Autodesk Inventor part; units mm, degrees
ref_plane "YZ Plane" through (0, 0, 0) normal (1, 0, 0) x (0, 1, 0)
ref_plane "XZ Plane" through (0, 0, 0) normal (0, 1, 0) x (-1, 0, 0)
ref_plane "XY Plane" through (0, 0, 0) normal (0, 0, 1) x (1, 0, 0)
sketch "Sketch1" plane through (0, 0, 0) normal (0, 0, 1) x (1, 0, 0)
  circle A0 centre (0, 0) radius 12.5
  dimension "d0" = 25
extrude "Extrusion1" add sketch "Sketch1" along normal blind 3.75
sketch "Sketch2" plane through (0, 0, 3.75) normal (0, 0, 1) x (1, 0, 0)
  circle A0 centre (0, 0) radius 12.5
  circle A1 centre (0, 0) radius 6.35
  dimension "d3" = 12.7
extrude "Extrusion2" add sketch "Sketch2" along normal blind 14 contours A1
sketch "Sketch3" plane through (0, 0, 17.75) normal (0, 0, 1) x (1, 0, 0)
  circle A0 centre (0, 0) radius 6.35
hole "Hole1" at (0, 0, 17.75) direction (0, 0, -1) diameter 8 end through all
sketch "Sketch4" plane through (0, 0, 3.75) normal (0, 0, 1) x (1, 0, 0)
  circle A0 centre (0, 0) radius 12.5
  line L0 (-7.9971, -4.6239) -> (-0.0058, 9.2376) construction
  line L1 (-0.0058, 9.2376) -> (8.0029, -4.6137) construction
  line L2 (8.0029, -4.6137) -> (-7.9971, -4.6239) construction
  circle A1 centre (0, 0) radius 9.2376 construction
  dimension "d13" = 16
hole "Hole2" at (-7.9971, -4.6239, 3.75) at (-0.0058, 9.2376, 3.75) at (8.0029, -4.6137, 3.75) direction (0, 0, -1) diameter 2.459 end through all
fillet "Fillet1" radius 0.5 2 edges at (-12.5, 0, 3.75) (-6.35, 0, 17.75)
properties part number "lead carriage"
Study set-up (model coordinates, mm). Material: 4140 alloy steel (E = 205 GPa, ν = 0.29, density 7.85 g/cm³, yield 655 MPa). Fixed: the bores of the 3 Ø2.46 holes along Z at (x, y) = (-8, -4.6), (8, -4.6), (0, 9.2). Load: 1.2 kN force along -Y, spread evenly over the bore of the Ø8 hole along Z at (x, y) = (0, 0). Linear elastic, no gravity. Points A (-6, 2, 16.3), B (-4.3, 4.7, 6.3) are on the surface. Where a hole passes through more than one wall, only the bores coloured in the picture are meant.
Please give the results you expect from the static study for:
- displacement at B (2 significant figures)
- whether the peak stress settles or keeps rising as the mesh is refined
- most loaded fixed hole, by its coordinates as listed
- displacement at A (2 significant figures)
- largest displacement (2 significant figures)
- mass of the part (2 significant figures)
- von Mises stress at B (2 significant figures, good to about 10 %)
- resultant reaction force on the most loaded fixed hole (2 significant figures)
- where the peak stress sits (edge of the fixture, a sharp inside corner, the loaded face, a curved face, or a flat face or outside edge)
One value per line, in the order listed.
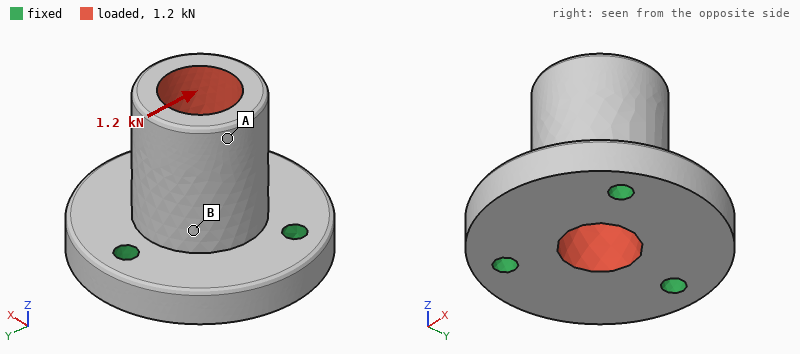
2.4 µm
keeps rising
(0, 9.2)
6.7 µm
7.9 µm
21 g
27 MPa
730 N
edge of the fixture
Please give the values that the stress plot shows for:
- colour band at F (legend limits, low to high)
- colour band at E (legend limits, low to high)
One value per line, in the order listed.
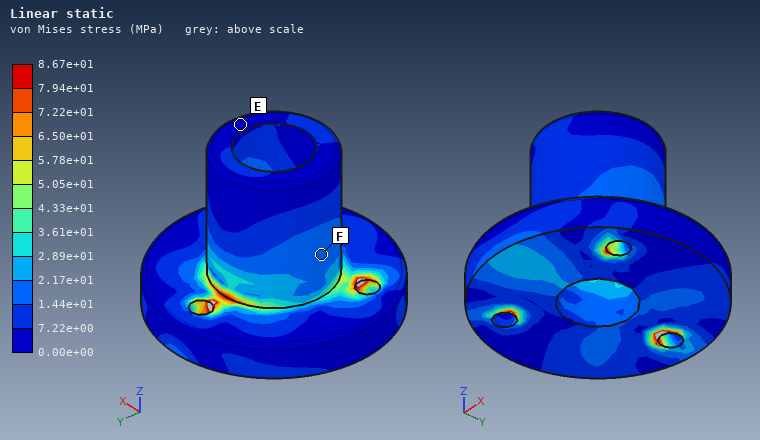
1.44e+01 to 2.17e+01 MPa
0.00e+00 to 7.22e+00 MPa
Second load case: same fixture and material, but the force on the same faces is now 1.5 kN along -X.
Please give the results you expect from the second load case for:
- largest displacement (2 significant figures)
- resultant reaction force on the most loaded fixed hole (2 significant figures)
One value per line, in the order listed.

9.8 µm
820 N
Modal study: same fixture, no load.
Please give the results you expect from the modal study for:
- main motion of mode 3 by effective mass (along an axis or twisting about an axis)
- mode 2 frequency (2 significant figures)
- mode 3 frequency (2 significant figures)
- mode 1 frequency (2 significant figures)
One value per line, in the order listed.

along Z
22 kHz
40 kHz
22 kHz
